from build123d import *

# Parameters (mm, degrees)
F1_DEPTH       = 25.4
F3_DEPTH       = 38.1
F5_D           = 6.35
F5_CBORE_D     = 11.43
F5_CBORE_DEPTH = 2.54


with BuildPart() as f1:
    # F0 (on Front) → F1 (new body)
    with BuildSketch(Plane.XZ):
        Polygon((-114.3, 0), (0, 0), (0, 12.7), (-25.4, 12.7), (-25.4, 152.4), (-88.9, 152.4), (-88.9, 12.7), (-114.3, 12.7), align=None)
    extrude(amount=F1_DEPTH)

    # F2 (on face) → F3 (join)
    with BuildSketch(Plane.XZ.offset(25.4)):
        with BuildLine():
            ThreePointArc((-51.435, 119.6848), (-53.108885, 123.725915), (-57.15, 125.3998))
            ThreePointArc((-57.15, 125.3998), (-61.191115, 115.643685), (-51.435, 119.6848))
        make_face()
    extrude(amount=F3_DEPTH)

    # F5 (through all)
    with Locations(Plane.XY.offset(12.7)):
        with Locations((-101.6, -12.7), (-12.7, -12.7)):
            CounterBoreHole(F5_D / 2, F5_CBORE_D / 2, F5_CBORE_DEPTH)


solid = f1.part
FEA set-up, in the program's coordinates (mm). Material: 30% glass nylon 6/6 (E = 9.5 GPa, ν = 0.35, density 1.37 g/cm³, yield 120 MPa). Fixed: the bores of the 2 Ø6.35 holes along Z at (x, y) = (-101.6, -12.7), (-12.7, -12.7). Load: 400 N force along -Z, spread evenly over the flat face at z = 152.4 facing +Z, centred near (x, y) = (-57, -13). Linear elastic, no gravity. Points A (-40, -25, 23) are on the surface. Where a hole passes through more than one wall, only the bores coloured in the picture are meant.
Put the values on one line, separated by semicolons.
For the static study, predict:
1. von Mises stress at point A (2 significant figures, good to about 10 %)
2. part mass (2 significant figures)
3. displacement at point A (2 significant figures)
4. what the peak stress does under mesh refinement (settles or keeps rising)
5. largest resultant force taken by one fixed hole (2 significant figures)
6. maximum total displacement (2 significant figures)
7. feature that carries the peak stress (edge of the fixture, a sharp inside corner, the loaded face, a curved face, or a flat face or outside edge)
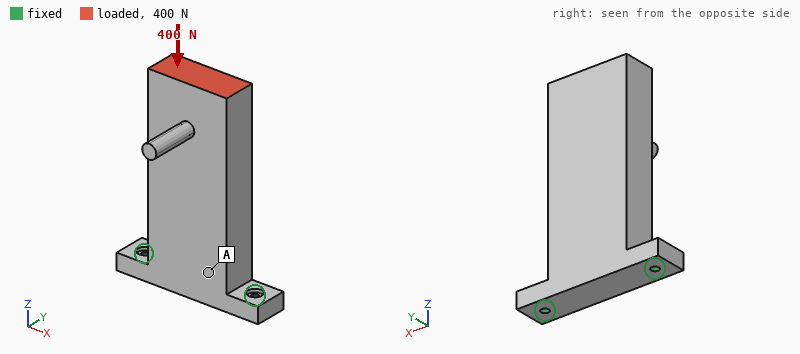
0.43 MPa; 360 g; 8.1 µm; keeps rising; 230 N; 11 µm; edge of the fixture
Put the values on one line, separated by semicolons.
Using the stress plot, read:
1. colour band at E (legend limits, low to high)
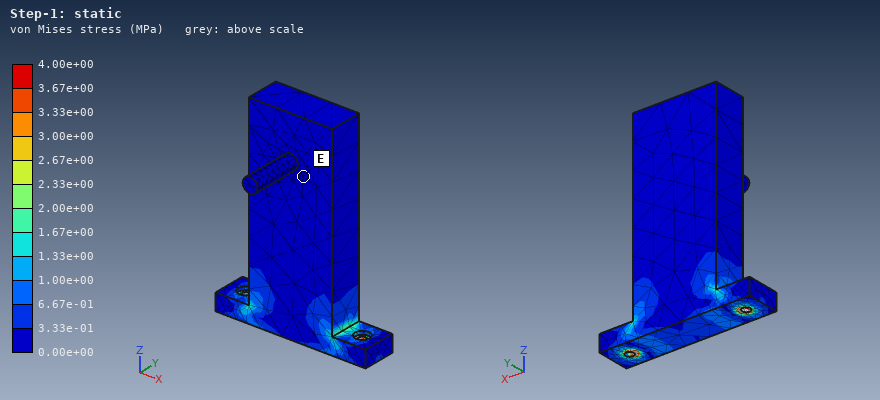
0.00e+00 to 3.33e-01 MPa
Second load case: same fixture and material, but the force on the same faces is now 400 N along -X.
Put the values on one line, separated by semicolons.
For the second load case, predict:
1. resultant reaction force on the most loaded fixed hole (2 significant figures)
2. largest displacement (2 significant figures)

790 N; 0.20 mm
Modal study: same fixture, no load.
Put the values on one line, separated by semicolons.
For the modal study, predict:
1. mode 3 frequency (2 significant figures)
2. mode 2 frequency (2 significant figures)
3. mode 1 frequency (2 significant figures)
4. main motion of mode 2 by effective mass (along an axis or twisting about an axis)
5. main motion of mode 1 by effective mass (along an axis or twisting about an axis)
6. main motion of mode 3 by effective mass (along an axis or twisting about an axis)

1600 Hz; 730 Hz; 200 Hz; along X; along Y; twisting about Z
